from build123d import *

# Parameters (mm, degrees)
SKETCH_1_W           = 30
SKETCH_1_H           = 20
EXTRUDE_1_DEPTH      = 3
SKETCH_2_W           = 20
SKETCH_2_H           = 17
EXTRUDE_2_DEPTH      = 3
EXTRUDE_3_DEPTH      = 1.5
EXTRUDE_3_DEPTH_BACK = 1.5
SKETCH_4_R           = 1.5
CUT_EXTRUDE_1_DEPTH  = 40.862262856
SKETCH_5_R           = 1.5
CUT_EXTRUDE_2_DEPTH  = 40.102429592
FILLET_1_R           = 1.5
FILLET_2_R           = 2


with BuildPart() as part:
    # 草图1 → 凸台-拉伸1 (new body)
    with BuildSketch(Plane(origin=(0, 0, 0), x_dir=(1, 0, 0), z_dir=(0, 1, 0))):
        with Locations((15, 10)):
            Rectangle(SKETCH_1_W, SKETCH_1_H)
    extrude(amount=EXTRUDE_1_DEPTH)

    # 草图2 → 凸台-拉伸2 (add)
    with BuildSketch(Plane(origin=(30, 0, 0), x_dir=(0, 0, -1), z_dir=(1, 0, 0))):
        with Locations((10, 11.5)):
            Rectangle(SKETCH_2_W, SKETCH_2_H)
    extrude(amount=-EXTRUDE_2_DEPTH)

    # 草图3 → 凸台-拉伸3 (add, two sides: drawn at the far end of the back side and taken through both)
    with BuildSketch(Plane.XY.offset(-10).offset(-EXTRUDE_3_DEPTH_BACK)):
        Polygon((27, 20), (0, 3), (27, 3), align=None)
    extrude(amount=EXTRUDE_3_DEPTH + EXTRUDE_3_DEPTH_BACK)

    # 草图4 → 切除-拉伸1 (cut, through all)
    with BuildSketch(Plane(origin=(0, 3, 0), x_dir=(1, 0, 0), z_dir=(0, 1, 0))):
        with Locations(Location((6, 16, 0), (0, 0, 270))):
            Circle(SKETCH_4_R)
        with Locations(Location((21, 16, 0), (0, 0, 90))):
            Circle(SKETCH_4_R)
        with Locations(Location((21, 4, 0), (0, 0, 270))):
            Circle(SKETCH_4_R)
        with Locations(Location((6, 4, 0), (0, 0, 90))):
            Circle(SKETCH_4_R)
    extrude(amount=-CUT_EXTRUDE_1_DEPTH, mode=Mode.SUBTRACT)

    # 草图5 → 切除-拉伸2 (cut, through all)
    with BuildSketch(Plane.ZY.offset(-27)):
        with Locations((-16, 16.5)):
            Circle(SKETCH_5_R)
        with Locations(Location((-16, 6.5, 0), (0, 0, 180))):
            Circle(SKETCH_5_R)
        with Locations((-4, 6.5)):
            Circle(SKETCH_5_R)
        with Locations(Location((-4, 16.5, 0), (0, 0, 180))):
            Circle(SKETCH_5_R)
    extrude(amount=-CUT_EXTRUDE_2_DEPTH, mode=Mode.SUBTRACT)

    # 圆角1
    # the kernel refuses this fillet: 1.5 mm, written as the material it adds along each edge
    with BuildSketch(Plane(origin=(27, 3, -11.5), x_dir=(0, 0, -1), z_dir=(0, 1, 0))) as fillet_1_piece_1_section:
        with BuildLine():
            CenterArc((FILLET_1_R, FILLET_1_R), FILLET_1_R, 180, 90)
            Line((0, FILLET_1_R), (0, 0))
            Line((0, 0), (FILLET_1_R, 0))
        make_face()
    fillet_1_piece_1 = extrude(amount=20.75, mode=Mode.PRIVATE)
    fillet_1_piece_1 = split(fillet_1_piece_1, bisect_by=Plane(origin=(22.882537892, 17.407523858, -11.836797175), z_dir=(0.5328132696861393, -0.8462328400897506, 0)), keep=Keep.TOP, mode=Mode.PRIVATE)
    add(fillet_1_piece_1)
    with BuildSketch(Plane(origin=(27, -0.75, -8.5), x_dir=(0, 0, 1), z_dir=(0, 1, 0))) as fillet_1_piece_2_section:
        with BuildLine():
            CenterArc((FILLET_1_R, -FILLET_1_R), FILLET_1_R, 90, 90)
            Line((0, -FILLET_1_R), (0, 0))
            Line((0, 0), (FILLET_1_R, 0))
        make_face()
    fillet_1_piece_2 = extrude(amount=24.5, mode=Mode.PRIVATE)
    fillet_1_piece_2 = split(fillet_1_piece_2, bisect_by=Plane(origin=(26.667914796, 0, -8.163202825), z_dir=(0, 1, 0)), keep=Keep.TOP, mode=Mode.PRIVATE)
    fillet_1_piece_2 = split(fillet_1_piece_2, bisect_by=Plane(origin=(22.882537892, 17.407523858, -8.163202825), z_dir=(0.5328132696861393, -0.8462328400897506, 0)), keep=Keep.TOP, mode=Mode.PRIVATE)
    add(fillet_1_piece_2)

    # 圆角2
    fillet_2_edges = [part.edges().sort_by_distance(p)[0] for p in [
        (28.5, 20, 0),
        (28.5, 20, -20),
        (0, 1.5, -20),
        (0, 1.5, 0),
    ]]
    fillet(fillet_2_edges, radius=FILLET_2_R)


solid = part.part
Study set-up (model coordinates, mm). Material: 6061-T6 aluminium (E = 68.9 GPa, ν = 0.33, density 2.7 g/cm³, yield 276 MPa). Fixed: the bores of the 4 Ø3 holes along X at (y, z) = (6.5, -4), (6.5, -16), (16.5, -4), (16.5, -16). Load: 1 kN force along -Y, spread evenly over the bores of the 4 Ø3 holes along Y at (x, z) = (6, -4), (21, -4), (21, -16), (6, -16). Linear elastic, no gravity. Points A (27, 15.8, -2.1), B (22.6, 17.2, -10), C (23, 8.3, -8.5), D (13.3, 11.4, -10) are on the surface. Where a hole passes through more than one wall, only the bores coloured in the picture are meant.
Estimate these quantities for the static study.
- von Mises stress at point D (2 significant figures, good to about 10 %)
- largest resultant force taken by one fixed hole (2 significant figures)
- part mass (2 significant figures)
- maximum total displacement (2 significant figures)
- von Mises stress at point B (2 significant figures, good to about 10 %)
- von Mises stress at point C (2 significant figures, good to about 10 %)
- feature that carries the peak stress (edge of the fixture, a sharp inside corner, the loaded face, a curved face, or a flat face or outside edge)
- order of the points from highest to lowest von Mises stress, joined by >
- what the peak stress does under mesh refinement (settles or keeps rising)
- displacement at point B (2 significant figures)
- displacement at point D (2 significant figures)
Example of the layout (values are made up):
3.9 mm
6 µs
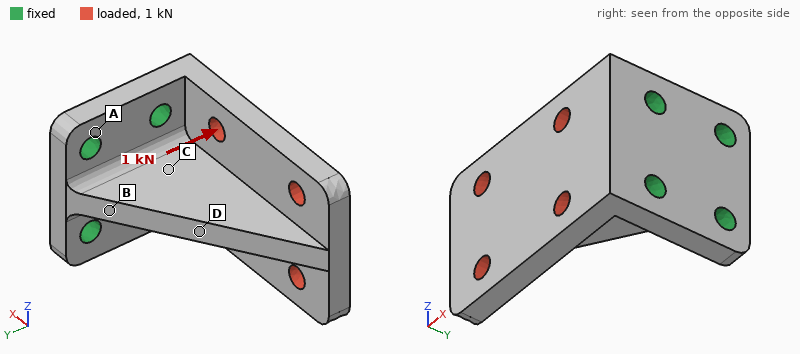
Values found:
50 MPa
620 N
9.0 g
85 µm
71 MPa
35 MPa
edge of the fixture
B > D > C > A
keeps rising
14 µm
35 µm
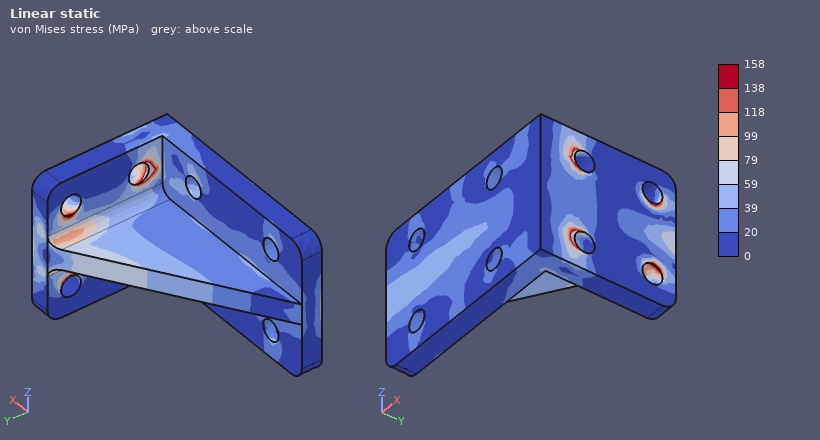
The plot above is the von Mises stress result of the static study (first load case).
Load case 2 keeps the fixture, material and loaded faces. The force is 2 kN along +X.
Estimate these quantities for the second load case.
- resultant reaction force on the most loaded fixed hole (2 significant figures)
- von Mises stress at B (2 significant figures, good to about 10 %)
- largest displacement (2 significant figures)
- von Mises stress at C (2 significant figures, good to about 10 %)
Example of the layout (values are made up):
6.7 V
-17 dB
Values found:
1.2 kN
37 MPa
56 µm
29 MPa
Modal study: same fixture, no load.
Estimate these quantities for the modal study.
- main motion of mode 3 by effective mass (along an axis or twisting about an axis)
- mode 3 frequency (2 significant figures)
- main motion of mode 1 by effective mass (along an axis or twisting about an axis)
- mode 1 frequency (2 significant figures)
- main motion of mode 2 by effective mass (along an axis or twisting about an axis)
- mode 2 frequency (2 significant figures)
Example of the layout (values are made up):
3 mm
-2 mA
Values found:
twisting about X
11 kHz
along Z
8500 Hz
along Y
9500 Hz
